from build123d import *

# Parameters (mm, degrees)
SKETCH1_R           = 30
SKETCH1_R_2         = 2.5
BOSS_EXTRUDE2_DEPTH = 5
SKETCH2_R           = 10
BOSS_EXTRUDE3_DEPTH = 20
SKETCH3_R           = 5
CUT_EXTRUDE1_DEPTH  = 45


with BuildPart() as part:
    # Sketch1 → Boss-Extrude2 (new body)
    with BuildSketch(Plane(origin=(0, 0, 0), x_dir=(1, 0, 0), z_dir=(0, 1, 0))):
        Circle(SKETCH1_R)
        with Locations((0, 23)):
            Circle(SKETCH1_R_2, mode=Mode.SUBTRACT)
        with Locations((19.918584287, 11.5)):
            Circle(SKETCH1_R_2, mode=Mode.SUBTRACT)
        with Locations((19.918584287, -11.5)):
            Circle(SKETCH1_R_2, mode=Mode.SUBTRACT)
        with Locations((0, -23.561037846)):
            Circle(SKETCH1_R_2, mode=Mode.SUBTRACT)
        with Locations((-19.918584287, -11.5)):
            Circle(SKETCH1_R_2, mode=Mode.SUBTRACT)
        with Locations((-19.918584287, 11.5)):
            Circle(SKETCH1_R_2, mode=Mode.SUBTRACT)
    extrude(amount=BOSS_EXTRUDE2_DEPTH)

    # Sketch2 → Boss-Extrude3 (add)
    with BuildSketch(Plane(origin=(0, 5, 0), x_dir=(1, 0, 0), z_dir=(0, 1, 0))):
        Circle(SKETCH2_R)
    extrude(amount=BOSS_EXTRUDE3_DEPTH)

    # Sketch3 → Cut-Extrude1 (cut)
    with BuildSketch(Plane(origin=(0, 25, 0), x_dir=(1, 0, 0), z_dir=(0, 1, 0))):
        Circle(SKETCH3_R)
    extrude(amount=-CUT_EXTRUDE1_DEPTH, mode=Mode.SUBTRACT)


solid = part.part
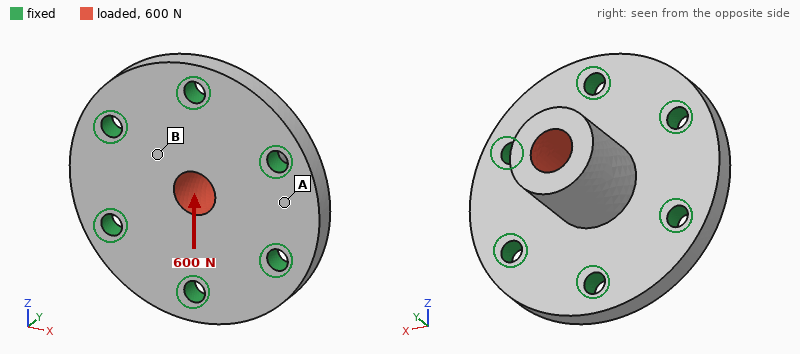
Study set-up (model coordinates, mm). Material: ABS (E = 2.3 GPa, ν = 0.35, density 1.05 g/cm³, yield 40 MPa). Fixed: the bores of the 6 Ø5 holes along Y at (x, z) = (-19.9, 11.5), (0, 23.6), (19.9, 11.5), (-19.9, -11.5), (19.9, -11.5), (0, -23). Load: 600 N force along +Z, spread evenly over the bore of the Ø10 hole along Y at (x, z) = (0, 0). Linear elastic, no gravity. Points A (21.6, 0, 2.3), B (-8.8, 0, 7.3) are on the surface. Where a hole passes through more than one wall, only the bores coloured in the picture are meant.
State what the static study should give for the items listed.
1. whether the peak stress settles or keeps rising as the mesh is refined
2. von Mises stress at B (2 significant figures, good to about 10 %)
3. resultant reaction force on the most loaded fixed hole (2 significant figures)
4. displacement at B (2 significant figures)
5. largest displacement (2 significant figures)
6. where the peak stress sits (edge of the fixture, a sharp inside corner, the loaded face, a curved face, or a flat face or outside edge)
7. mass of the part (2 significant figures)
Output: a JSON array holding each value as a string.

["keeps rising", "4.5 MPa", "200 N", "0.039 mm", "0.25 mm", "edge of the fixture", "19 g"]
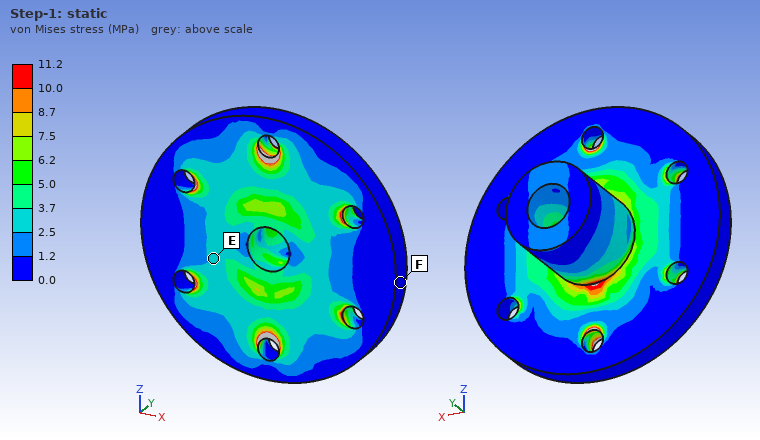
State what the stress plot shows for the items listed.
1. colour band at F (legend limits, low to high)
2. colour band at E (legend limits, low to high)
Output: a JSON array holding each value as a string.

["0.0 to 1.2 MPa", "2.5 to 3.7 MPa"]
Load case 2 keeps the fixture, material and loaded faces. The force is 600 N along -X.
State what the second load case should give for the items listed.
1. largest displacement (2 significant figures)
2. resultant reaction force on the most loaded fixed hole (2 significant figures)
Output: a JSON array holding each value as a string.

["0.24 mm", "170 N"]
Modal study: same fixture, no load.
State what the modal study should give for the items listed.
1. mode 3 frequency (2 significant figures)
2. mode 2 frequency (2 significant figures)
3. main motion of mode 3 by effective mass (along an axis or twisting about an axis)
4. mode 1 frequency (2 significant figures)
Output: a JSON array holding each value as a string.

["4400 Hz", "3700 Hz", "along Y", "3600 Hz"]
